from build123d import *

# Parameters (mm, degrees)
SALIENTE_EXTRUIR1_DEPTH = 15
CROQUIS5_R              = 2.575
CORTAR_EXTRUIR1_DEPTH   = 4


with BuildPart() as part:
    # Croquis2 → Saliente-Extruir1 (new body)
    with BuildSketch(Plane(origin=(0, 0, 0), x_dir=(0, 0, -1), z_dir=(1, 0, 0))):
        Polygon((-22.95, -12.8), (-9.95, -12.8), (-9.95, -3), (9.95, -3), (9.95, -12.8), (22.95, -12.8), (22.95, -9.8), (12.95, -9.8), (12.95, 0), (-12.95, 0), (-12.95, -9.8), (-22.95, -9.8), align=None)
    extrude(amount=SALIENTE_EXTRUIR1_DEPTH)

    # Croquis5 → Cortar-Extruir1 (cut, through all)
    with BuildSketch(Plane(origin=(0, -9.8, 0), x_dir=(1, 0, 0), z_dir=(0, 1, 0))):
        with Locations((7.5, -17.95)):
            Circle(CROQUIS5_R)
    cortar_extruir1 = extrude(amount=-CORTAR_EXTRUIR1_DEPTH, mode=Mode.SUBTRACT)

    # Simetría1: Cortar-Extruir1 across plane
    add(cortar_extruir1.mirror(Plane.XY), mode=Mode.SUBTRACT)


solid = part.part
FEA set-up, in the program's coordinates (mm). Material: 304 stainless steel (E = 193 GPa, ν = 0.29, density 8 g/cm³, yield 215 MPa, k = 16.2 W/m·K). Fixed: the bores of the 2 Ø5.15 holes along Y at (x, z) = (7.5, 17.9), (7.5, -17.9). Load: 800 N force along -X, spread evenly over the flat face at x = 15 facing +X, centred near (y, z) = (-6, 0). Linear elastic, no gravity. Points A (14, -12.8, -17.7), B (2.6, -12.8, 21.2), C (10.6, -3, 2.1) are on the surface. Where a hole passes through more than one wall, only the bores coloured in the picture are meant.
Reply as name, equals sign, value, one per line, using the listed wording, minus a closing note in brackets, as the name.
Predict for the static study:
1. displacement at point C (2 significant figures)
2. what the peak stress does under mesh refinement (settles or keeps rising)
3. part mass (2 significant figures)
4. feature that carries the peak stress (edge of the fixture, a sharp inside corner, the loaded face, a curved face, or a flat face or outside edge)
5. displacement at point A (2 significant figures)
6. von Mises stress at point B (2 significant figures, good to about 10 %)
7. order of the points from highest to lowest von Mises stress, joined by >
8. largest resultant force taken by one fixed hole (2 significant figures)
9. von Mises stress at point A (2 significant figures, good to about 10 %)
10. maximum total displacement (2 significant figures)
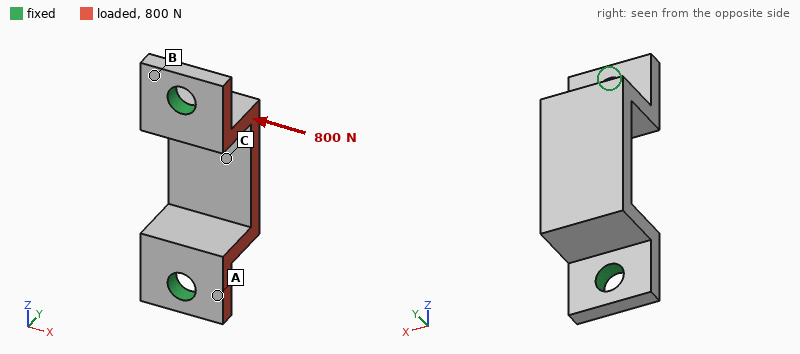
displacement at point C = 7.6 µm
what the peak stress does under mesh refinement = keeps rising
part mass = 23 g
feature that carries the peak stress = edge of the fixture
displacement at point A = 1.6 µm
von Mises stress at point B = 19 MPa
order of the points from highest to lowest von Mises stress, joined by > = A > B > C
largest resultant force taken by one fixed hole = 400 N
von Mises stress at point A = 29 MPa
maximum total displacement = 11 µm
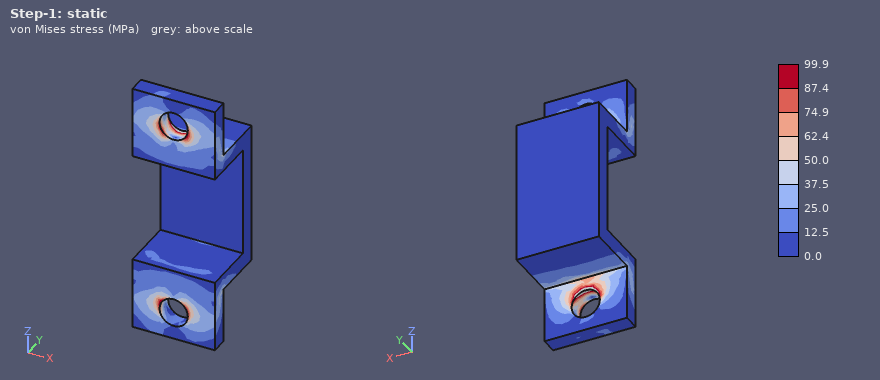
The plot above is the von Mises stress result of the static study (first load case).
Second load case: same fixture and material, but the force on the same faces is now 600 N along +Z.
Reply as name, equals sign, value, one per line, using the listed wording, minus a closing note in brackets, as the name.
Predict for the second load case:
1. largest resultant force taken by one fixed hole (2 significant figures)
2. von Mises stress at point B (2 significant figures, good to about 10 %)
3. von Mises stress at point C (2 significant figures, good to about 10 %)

largest resultant force taken by one fixed hole = 320 N
von Mises stress at point B = 5.6 MPa
von Mises stress at point C = 17 MPa
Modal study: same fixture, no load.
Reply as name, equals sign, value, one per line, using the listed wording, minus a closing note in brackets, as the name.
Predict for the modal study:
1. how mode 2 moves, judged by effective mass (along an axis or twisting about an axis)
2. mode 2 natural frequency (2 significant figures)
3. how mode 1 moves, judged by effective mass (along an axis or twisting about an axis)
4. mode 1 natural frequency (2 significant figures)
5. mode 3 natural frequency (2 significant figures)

how mode 2 moves, judged by effective mass = along Z
mode 2 natural frequency = 12 kHz
how mode 1 moves, judged by effective mass = along X
mode 1 natural frequency = 9800 Hz
mode 3 natural frequency = 15 kHz
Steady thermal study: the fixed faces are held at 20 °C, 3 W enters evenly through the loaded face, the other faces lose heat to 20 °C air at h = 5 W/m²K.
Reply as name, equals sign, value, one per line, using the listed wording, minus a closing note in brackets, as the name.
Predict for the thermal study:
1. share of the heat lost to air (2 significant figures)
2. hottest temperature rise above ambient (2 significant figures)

share of the heat lost to air = 4.0 %
hottest temperature rise above ambient = 24 K
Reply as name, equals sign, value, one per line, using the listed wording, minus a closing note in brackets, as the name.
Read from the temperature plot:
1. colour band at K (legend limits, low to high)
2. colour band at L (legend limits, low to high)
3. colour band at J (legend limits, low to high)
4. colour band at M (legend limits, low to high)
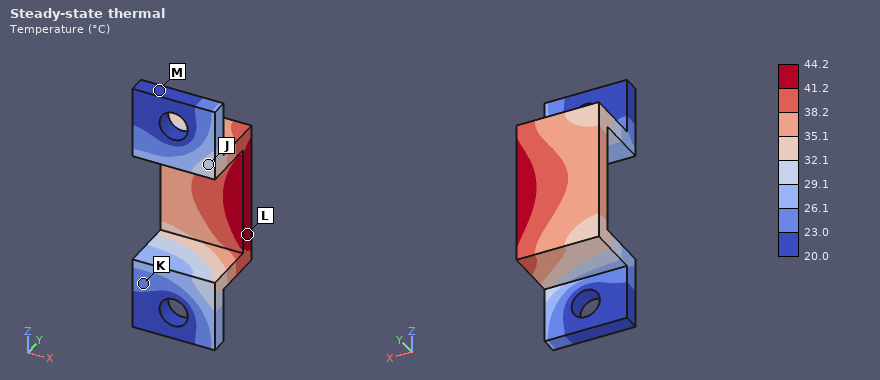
colour band at K = 23.0 to 26.1 °C
colour band at L = 41.2 to 44.2 °C
colour band at J = 29.1 to 32.1 °C
colour band at M = 20.0 to 23.0 °C
